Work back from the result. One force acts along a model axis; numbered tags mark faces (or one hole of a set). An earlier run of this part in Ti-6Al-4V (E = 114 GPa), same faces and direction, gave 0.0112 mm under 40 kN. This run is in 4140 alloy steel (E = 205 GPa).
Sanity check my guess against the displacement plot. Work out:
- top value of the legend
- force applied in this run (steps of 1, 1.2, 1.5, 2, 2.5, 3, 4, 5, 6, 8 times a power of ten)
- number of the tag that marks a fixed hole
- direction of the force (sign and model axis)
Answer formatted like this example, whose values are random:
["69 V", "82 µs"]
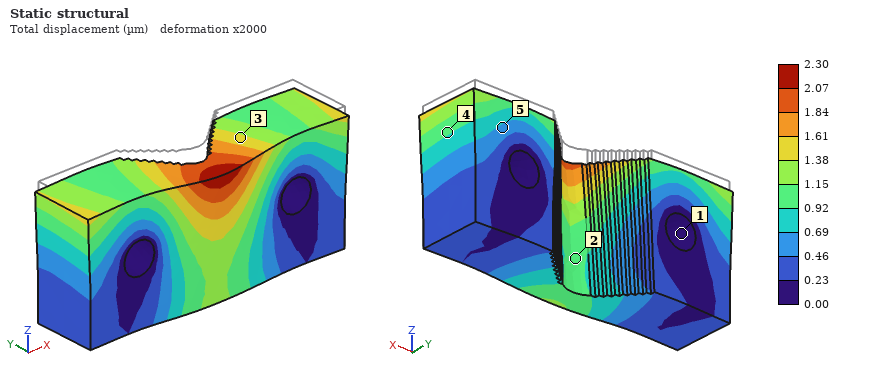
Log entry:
["2.30 µm", "15 kN", "1", "-Z"]
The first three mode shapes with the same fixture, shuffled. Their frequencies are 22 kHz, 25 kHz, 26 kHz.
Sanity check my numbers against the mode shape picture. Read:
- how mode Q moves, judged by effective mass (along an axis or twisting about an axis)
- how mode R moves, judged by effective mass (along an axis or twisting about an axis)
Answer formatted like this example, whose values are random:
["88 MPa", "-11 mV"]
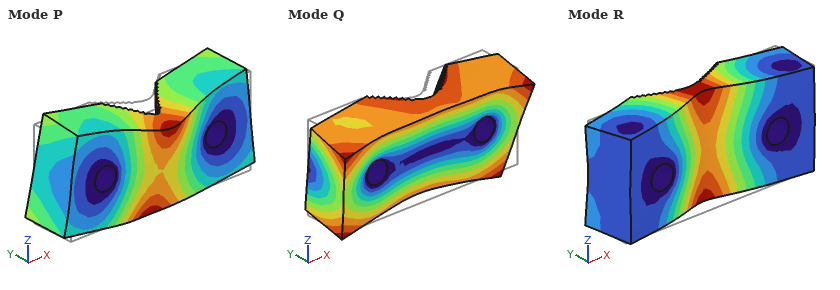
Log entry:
["twisting about X", "along Y"]
